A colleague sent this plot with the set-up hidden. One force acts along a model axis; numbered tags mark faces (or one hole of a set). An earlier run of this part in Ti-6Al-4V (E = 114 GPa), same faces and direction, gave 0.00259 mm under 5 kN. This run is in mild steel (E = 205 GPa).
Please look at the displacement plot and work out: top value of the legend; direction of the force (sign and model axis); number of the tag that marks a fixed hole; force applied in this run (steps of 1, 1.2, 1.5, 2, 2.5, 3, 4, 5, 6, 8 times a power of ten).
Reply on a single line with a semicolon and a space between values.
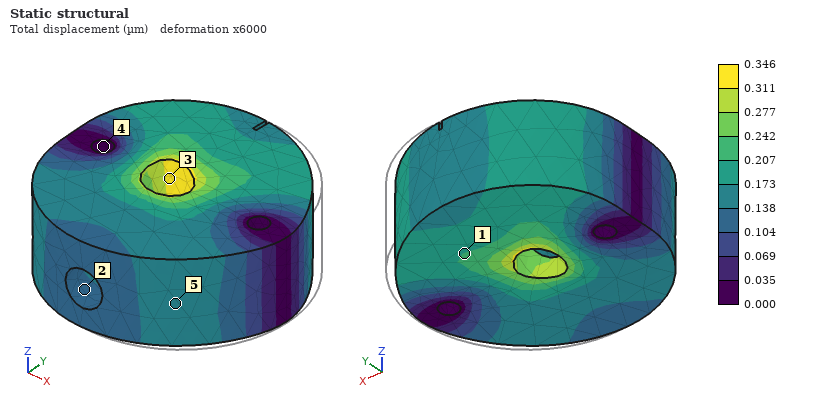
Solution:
0.346 µm; -X; 4; 1.2 kN
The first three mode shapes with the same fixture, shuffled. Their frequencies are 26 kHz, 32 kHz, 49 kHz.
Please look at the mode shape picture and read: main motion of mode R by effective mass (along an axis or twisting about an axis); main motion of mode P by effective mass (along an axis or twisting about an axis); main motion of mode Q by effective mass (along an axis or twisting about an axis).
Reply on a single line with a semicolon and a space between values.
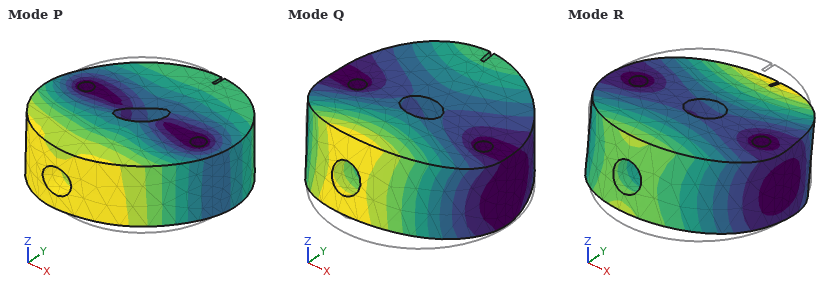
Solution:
twisting about X; twisting about Z; along Z
